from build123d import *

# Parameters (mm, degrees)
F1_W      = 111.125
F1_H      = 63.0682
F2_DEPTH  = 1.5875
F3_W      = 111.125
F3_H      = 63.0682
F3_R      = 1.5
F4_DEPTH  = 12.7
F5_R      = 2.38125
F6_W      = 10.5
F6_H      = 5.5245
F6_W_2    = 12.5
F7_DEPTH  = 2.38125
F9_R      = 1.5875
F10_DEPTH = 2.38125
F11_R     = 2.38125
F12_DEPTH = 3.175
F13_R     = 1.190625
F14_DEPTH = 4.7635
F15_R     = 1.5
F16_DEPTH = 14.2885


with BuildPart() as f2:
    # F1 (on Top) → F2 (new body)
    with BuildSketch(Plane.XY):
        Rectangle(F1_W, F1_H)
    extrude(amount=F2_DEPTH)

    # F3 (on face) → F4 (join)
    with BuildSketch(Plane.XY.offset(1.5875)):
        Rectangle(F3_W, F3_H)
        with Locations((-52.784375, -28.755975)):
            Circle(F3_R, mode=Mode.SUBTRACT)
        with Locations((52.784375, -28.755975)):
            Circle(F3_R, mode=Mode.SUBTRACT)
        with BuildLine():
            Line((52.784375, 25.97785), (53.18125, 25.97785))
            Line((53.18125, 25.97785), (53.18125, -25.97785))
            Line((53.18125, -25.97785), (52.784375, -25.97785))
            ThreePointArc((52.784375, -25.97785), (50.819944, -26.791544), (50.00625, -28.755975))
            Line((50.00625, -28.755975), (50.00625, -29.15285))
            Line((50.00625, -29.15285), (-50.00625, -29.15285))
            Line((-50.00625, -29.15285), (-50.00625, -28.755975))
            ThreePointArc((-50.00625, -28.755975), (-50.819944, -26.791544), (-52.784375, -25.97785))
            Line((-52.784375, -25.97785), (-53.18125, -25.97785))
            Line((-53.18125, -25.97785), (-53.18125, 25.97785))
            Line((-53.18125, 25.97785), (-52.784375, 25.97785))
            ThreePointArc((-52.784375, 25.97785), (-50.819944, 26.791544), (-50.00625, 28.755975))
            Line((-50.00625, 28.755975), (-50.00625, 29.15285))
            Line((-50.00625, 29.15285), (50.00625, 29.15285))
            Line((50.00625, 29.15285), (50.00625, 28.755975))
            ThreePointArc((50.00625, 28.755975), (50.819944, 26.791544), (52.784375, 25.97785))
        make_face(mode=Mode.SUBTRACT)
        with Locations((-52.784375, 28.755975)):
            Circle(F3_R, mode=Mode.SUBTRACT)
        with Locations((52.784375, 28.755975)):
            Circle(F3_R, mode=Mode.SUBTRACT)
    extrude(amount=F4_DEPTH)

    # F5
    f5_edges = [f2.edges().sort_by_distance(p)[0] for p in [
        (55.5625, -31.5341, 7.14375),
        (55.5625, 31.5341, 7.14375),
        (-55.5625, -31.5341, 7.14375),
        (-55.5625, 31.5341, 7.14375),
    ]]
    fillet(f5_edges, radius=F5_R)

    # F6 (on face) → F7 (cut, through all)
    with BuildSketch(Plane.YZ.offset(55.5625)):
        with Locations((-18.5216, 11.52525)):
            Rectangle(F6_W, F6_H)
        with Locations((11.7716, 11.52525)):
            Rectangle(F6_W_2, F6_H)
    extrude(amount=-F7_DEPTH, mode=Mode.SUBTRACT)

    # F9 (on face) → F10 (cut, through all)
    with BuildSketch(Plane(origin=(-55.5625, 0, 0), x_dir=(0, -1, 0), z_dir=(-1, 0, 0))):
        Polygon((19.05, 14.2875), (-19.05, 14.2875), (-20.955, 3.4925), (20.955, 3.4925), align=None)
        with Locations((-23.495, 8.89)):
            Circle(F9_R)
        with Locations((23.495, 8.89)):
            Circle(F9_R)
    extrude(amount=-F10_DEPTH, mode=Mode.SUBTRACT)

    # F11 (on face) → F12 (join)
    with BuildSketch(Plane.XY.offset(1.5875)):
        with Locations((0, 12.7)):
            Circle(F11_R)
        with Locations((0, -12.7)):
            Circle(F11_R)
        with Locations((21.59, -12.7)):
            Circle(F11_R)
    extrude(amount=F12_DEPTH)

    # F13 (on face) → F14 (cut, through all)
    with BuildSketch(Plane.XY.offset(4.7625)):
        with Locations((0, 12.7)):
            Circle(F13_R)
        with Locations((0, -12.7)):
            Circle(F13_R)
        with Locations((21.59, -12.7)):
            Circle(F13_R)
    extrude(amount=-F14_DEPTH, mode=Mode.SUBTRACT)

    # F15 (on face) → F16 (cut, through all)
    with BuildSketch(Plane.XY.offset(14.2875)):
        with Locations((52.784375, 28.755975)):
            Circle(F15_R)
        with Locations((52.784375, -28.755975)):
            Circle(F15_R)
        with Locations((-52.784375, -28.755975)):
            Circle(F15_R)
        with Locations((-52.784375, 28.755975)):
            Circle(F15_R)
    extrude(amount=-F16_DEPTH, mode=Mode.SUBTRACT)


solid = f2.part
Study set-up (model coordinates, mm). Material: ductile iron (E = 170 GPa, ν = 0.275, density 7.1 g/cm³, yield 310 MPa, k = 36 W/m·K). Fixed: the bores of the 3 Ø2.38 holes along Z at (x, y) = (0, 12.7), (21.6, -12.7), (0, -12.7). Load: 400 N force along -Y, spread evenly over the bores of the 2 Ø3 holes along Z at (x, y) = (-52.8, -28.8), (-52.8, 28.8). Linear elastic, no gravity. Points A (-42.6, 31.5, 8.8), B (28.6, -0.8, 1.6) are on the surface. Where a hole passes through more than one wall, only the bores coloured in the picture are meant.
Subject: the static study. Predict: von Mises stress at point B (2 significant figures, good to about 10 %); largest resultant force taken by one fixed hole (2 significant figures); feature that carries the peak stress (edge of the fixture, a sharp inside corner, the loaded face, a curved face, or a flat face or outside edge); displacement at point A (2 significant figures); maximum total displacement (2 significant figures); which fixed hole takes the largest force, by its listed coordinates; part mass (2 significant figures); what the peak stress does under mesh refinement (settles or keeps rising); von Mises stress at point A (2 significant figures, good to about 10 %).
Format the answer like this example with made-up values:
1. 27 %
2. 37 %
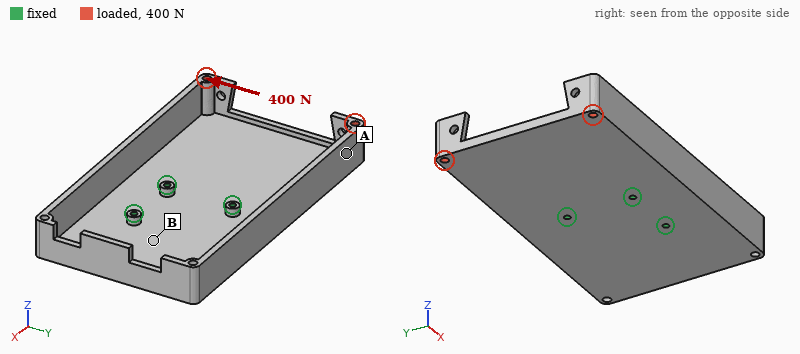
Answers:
1. 8.7 MPa
2. 660 N
3. edge of the fixture
4. 0.15 mm
5. 0.19 mm
6. (0, 12.7)
7. 140 g
8. keeps rising
9. 22 MPa
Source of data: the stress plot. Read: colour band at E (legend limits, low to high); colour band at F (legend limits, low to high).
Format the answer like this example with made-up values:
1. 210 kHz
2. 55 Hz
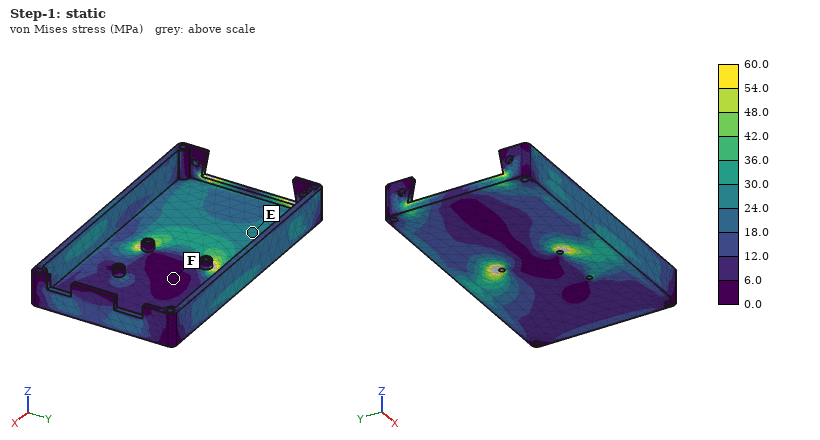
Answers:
1. 24.0 to 30.0 MPa
2. 0.0 to 6.0 MPa
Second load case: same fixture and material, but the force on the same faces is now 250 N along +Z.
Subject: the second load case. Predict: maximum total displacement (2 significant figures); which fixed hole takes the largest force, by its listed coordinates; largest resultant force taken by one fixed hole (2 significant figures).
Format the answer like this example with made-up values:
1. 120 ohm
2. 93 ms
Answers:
1. 0.70 mm
2. (0, -12.7)
3. 420 N
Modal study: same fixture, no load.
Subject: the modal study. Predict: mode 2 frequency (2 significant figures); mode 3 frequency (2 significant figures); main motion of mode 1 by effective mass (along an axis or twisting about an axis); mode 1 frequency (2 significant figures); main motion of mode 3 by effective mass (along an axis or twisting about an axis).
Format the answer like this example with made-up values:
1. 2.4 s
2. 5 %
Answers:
1. 760 Hz
2. 920 Hz
3. twisting about Y
4. 490 Hz
5. along Z
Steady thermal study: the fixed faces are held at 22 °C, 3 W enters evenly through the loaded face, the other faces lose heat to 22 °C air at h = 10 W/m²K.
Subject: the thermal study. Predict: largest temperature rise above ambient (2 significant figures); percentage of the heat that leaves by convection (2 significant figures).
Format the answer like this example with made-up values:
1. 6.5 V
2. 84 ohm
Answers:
1. 27 K
2. 53 %
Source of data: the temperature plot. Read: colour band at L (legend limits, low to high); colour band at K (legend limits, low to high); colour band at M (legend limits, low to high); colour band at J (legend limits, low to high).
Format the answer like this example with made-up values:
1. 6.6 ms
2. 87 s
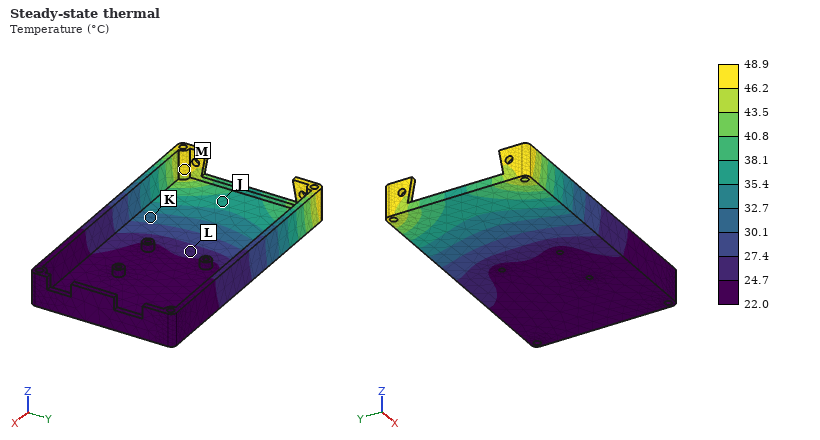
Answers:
1. 24.7 to 27.4 °C
2. 30.1 to 32.7 °C
3. 46.2 to 48.9 °C
4. 35.4 to 38.1 °C
